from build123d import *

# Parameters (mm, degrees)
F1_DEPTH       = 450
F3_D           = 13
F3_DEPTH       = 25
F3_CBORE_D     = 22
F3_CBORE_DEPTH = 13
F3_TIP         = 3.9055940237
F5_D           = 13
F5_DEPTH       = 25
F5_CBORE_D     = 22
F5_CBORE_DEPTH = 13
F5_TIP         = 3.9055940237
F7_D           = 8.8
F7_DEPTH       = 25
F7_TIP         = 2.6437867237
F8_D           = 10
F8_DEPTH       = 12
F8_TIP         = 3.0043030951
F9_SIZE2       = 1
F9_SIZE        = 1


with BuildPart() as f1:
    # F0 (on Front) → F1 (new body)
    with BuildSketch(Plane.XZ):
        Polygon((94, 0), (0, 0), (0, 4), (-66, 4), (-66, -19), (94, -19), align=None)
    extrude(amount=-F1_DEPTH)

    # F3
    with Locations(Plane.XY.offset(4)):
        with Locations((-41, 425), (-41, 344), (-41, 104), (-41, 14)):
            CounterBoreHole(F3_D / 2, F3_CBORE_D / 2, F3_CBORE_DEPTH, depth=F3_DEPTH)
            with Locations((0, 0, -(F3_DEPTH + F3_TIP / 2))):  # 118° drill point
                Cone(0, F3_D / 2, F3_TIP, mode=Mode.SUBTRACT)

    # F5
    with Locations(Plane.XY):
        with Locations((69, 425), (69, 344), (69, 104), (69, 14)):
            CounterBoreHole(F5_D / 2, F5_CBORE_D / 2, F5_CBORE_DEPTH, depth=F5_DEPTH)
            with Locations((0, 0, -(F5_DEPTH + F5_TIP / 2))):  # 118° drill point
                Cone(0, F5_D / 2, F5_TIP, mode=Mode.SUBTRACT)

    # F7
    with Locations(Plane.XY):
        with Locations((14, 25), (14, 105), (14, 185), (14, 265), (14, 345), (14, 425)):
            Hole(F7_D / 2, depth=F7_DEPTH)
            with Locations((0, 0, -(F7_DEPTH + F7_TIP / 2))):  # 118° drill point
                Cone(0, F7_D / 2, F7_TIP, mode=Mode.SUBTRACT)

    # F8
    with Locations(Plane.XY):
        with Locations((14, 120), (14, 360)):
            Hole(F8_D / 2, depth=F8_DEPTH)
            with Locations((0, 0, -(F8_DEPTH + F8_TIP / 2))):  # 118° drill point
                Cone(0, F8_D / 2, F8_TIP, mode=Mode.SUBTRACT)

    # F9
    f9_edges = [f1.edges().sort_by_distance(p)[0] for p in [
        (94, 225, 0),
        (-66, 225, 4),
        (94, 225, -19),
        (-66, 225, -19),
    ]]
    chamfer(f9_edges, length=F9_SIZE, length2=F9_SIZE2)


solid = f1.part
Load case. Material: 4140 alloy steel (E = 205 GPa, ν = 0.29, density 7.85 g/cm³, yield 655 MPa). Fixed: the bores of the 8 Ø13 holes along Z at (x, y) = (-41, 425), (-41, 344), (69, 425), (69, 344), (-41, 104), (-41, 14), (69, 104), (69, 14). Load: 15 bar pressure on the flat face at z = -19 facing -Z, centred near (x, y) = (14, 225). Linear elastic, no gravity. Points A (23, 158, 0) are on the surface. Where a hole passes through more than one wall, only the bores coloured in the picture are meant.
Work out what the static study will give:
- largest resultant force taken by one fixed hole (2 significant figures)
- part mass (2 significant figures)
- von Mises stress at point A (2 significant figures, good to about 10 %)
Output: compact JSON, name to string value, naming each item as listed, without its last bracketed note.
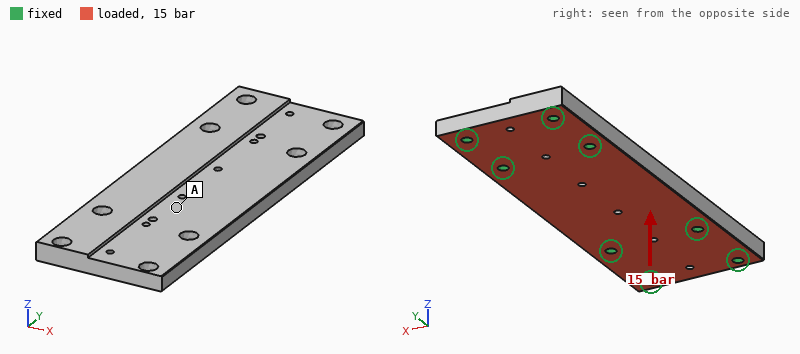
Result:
{"largest resultant force taken by one fixed hole": "27 kN", "part mass": "11 kg", "von Mises stress at point A": "26 MPa"}
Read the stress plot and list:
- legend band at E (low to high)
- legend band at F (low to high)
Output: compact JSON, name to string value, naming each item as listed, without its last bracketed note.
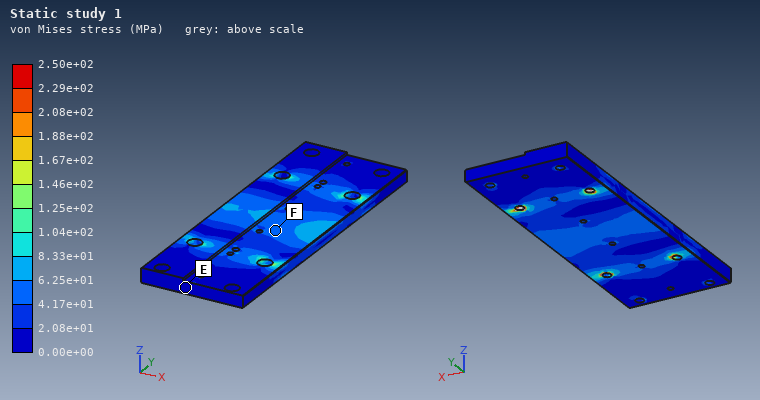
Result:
{"legend band at E": "0.00e+00 to 2.08e+01 MPa", "legend band at F": "4.17e+01 to 6.25e+01 MPa"}
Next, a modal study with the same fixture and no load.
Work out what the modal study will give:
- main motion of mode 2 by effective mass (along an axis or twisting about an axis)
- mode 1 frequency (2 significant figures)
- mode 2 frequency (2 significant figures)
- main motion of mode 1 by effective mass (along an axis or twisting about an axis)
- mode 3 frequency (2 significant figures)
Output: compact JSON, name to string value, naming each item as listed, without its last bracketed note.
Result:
{"main motion of mode 2 by effective mass": "twisting about Y", "mode 1 frequency": "1500 Hz", "mode 2 frequency": "2200 Hz", "main motion of mode 1 by effective mass": "along Z", "mode 3 frequency": "3700 Hz"}
